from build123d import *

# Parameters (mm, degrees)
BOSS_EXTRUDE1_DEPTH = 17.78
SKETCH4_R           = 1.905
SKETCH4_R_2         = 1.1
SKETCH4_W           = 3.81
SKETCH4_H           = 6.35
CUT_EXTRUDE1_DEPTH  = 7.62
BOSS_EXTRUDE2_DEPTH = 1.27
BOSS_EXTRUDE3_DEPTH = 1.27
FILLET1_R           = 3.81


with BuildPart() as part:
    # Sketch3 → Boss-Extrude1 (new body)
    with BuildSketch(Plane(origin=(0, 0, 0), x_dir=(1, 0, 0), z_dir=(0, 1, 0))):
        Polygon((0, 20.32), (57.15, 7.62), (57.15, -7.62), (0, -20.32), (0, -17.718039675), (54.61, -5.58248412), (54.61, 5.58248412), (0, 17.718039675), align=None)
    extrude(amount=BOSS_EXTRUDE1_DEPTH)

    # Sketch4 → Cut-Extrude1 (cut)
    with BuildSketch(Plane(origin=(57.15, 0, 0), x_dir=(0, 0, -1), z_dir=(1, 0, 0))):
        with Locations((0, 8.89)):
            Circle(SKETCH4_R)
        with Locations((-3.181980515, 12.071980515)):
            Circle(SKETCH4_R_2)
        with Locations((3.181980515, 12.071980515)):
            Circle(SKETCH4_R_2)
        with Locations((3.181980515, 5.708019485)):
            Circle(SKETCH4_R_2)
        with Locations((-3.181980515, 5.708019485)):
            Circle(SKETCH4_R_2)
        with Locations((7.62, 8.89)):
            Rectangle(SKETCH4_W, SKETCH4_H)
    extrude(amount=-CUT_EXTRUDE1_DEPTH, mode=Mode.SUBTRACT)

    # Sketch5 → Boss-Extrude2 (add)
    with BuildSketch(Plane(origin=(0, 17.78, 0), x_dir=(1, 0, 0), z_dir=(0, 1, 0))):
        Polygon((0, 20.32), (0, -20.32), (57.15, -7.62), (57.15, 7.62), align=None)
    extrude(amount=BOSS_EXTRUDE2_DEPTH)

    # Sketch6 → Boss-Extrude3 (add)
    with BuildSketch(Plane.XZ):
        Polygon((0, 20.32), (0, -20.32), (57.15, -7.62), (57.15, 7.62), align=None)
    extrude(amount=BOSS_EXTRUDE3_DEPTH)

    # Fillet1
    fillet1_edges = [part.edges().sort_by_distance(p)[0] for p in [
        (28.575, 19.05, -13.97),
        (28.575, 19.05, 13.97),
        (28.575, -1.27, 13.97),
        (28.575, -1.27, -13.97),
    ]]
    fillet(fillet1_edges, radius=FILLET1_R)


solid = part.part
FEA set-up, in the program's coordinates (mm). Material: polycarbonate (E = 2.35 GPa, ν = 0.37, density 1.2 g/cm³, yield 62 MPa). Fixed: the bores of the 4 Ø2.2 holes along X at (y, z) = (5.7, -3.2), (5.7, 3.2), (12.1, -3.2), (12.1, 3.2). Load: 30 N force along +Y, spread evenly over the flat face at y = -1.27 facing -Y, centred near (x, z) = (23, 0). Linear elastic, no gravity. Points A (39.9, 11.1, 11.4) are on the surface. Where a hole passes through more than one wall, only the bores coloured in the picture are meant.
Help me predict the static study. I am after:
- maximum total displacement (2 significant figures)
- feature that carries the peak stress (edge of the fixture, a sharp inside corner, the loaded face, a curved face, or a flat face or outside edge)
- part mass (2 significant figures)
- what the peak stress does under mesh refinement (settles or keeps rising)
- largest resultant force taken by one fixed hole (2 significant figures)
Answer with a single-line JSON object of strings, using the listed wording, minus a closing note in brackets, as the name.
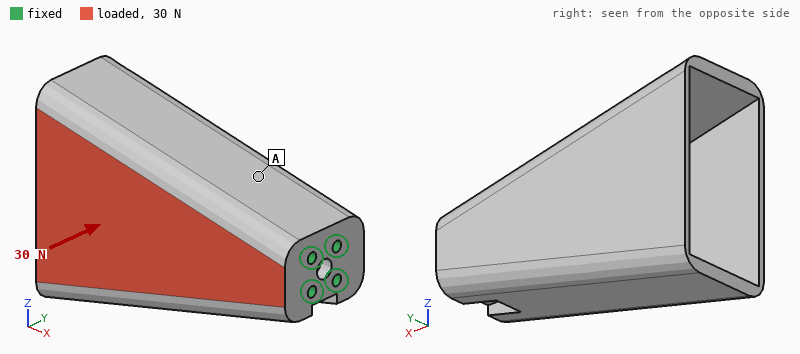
{"maximum total displacement": "0.70 mm", "feature that carries the peak stress": "edge of the fixture", "part mass": "11 g", "what the peak stress does under mesh refinement": "keeps rising", "largest resultant force taken by one fixed hole": "54 N"}
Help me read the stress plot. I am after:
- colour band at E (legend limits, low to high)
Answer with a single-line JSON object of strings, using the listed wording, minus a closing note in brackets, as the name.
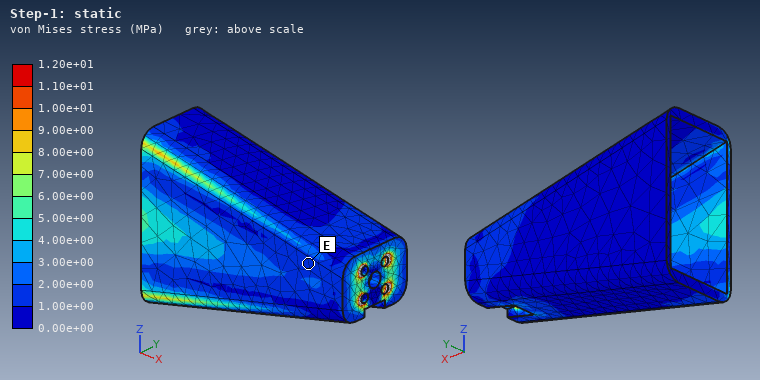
{"colour band at E": "1.00e+00 to 2.00e+00 MPa"}
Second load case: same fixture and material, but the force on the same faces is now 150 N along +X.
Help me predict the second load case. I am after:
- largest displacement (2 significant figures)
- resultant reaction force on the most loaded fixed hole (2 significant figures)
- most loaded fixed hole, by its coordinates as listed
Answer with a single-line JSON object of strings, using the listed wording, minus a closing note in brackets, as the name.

{"largest displacement": "0.71 mm", "resultant reaction force on the most loaded fixed hole": "120 N", "most loaded fixed hole, by its coordinates as listed": "(5.7, 3.2)"}
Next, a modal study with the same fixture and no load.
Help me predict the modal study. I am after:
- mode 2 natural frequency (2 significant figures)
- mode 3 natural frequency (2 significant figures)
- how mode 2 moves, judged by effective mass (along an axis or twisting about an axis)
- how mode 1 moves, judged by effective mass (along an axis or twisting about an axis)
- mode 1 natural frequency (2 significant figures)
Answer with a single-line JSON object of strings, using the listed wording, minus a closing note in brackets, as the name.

{"mode 2 natural frequency": "540 Hz", "mode 3 natural frequency": "1000 Hz", "how mode 2 moves, judged by effective mass": "along Y", "how mode 1 moves, judged by effective mass": "along Z", "mode 1 natural frequency": "510 Hz"}
